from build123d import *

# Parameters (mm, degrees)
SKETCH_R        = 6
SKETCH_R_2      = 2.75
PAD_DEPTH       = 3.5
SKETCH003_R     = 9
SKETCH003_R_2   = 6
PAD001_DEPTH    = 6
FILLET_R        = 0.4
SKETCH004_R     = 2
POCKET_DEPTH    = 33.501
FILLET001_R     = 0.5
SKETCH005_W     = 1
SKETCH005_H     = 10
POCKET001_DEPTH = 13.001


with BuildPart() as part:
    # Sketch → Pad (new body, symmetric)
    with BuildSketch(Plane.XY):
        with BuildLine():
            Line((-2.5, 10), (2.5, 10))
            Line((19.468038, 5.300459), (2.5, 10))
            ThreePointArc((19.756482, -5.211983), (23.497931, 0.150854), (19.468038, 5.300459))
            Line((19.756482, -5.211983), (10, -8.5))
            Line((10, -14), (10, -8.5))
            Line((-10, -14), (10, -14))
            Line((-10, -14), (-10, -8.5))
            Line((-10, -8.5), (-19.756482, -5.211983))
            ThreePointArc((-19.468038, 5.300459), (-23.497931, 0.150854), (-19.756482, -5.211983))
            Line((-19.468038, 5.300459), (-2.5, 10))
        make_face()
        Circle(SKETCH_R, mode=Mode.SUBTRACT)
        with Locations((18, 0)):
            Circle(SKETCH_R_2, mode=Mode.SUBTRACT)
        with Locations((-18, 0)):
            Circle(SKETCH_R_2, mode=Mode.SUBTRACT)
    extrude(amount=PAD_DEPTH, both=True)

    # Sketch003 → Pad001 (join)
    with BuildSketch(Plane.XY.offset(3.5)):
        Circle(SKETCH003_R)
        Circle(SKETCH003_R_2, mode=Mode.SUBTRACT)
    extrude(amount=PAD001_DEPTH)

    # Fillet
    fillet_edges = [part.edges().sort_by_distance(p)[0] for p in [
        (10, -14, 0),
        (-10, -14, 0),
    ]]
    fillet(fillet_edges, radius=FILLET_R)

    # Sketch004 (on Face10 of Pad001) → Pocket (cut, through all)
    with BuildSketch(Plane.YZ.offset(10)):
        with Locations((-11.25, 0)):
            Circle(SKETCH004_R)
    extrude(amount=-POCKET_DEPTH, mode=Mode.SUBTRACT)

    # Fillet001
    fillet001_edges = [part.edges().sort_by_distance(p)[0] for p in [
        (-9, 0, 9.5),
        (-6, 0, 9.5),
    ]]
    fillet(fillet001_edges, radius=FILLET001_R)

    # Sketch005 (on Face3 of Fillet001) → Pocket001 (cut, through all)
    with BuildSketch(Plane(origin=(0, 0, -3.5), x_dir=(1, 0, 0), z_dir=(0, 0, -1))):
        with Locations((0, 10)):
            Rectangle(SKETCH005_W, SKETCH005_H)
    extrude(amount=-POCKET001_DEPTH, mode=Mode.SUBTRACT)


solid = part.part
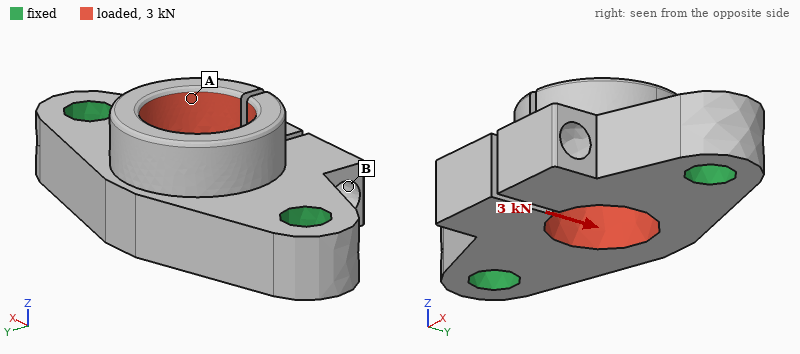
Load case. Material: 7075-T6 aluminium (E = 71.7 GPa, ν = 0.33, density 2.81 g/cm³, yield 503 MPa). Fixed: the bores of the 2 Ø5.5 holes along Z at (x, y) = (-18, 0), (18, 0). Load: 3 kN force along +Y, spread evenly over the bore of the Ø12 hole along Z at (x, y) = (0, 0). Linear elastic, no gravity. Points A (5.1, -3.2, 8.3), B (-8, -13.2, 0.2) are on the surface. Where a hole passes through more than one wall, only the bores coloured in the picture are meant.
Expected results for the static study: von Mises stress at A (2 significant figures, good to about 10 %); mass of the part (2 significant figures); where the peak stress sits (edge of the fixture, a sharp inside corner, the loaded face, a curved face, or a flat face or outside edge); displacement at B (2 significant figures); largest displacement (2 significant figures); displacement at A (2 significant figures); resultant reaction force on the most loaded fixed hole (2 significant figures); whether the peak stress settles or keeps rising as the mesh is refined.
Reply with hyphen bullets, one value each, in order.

- 34 MPa
- 14 g
- edge of the fixture
- 27 µm
- 45 µm
- 29 µm
- 1.9 kN
- keeps rising
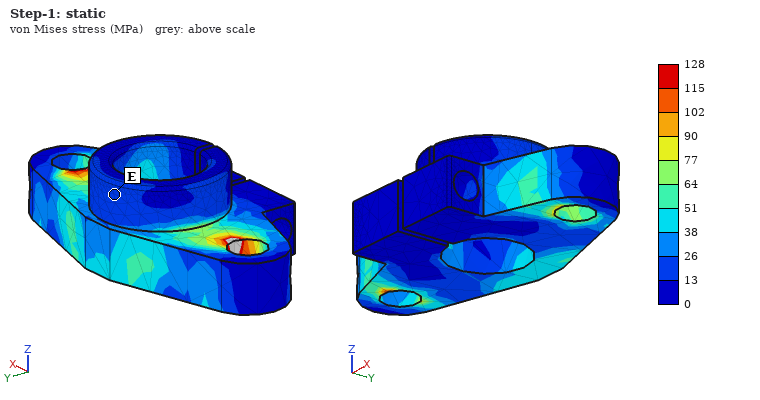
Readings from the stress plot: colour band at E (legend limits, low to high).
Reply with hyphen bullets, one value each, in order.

- 13 to 26 MPa
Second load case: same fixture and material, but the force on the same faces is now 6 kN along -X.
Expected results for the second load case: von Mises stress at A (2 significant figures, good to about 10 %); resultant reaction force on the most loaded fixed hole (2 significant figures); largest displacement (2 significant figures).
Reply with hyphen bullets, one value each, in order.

- 13 MPa
- 3.0 kN
- 39 µm
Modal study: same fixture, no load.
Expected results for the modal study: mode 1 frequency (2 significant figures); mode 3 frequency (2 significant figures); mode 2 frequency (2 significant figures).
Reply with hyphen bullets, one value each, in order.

- 16 kHz
- 19 kHz
- 16 kHz
